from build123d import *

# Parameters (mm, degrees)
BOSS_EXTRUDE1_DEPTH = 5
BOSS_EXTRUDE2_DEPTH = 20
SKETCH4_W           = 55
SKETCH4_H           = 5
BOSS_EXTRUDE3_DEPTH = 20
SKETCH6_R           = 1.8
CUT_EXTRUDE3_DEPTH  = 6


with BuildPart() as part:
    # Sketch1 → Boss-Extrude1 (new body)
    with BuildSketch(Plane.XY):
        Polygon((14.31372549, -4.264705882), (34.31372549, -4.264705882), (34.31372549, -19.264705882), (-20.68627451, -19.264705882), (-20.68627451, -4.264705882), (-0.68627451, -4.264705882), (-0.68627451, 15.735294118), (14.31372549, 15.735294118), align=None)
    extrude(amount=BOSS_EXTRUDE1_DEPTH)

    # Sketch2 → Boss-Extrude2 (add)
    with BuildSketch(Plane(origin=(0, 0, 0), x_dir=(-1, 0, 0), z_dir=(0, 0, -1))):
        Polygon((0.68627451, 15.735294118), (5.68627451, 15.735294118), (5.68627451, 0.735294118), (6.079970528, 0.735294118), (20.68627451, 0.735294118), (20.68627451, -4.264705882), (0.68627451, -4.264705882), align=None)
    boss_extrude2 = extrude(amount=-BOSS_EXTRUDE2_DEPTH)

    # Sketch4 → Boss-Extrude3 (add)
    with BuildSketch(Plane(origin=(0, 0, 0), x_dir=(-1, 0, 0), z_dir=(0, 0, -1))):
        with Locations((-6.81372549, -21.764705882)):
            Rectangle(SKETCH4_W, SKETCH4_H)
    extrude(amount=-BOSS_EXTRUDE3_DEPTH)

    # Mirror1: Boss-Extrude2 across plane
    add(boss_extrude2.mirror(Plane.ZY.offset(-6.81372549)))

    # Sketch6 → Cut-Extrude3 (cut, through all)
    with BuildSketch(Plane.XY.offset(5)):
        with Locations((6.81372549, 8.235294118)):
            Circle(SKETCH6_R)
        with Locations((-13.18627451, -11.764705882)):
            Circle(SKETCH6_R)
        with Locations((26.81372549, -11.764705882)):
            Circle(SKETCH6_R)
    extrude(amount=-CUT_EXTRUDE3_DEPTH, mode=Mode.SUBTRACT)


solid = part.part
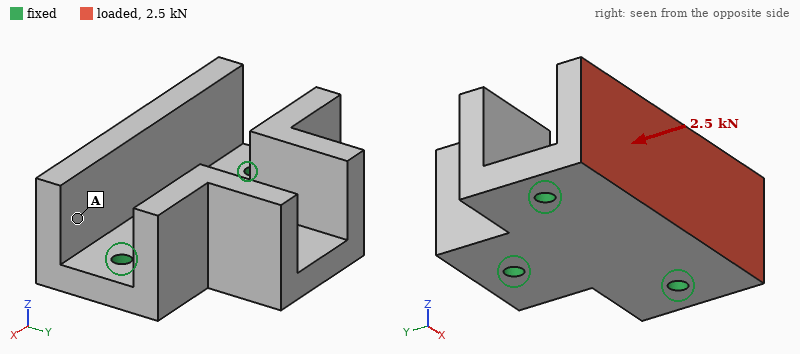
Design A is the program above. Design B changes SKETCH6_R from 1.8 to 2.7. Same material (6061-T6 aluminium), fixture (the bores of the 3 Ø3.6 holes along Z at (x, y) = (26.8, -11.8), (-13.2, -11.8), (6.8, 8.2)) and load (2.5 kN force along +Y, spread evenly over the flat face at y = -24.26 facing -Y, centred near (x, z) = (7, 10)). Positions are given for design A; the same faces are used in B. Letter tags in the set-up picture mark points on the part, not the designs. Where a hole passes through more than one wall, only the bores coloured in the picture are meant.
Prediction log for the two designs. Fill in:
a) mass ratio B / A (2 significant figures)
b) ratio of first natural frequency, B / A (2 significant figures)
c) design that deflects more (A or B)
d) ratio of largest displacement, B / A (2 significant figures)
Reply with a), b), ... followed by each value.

a) 0.99
b) 1.1
c) A
d) 0.89
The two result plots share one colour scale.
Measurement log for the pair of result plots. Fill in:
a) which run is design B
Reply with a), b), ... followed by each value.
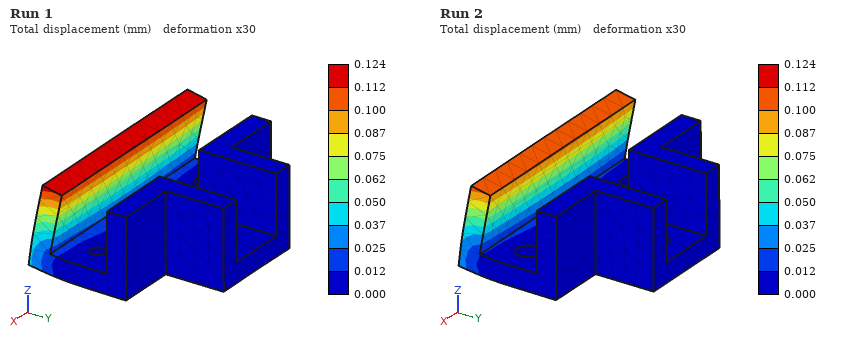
a) Run 2
